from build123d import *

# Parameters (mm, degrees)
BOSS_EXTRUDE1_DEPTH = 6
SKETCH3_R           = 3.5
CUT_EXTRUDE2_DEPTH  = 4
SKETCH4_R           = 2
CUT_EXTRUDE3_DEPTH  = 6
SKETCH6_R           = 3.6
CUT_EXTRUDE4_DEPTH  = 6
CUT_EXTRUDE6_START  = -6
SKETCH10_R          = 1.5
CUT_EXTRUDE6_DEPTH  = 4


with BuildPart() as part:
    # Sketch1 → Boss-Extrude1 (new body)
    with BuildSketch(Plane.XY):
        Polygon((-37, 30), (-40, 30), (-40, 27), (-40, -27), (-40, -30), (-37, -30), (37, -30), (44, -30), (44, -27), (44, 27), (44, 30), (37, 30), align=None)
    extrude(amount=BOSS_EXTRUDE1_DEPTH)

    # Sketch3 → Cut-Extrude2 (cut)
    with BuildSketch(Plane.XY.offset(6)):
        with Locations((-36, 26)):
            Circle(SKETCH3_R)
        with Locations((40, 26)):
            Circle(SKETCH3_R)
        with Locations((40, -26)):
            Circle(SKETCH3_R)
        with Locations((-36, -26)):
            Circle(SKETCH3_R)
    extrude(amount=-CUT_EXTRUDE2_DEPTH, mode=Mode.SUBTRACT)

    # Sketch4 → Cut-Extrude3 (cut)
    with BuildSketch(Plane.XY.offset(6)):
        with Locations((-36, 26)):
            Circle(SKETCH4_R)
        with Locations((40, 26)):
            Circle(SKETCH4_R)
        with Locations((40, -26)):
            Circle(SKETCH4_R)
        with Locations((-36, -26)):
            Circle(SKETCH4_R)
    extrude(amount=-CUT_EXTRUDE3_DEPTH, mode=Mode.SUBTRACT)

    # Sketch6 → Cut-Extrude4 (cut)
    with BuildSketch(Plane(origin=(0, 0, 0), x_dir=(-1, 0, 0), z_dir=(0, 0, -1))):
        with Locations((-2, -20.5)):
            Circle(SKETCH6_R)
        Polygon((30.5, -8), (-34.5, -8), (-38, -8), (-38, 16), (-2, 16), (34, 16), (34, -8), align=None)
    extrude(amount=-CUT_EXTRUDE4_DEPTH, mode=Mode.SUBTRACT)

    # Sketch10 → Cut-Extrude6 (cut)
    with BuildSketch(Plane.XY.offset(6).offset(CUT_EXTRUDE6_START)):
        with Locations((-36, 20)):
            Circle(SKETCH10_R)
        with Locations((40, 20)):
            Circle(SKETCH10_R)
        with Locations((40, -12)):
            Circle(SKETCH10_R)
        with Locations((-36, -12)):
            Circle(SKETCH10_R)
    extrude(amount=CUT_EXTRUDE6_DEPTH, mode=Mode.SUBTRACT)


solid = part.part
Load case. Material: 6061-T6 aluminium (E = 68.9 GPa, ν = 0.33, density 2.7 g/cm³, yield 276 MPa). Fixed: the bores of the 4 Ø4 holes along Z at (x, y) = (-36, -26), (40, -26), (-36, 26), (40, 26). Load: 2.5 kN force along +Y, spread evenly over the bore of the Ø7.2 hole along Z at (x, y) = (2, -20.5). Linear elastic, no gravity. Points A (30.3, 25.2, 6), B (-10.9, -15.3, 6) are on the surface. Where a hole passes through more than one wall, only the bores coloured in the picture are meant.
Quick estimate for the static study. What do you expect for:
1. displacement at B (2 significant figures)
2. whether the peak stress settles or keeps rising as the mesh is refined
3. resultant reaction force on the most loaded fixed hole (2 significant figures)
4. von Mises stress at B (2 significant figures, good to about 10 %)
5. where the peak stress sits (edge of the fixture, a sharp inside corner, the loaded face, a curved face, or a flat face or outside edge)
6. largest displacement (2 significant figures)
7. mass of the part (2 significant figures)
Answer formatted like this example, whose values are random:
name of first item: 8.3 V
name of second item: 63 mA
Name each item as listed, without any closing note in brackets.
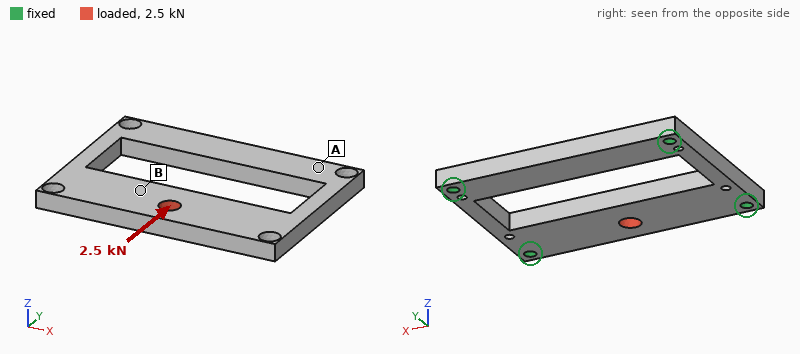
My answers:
displacement at B: 57 µm
whether the peak stress settles or keeps rising as the mesh is refined: keeps rising
resultant reaction force on the most loaded fixed hole: 1.5 kN
von Mises stress at B: 25 MPa
where the peak stress sits: edge of the fixture
largest displacement: 70 µm
mass of the part: 51 g
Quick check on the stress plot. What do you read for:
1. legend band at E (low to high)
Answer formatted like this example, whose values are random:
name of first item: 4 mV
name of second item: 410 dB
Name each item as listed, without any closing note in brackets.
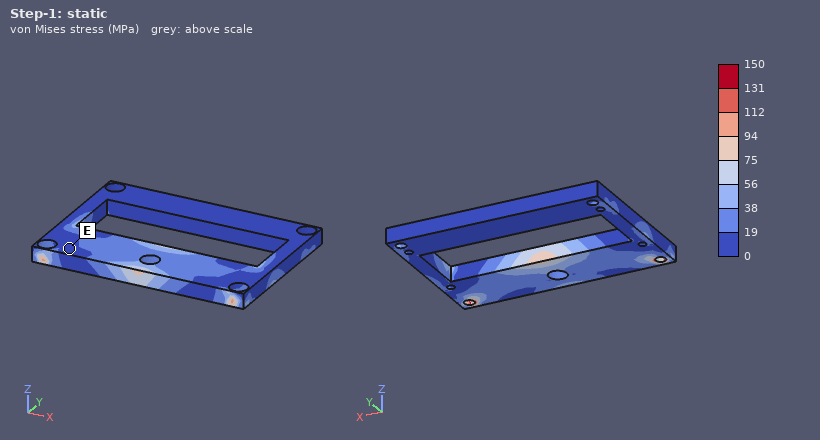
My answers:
legend band at E: 0 to 19 MPa
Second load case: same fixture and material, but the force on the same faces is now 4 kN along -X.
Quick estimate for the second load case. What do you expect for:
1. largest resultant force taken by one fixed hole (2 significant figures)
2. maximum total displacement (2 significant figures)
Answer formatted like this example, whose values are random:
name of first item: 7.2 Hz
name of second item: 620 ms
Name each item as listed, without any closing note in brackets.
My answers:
largest resultant force taken by one fixed hole: 2.0 kN
maximum total displacement: 21 µm
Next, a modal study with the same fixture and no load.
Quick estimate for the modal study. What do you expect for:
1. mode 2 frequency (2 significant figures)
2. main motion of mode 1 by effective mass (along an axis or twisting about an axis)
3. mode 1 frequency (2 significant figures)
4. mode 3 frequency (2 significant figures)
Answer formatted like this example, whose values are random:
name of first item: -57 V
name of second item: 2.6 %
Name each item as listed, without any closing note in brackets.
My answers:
mode 2 frequency: 3900 Hz
main motion of mode 1 by effective mass: along Z
mode 1 frequency: 3300 Hz
mode 3 frequency: 6800 Hz
